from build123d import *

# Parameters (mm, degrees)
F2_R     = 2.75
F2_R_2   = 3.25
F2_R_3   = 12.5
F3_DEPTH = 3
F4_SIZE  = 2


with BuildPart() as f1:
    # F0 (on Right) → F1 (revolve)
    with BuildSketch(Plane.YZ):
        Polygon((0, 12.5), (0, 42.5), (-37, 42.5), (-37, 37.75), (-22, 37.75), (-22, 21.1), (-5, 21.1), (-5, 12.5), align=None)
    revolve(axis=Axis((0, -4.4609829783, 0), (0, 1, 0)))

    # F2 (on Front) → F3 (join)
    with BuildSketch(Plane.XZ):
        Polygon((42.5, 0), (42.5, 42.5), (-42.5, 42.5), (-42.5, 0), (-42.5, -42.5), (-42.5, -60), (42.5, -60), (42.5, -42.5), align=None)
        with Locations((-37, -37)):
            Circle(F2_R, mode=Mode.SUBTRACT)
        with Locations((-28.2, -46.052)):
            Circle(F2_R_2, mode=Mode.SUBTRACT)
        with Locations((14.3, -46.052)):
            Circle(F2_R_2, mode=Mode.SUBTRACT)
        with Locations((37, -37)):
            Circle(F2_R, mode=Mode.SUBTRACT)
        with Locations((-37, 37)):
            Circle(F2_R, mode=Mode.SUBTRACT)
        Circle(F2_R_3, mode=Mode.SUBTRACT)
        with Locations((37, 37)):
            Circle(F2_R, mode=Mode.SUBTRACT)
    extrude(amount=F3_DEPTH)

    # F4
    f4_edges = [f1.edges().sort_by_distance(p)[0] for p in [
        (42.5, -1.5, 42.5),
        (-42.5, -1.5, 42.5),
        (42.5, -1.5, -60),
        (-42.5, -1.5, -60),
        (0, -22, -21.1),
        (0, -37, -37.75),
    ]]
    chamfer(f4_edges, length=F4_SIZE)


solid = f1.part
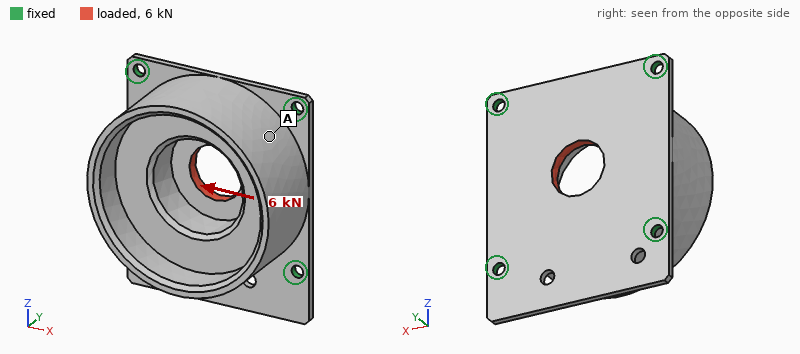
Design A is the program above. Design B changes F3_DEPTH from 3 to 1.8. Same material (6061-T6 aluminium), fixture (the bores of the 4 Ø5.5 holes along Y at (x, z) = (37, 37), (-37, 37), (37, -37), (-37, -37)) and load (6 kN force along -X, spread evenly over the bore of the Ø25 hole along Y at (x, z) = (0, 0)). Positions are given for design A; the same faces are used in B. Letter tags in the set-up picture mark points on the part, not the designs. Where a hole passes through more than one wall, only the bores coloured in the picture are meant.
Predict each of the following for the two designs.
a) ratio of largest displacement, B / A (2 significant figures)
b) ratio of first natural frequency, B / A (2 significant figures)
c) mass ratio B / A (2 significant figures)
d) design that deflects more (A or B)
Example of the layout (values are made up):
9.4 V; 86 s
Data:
1.3; 0.58; 0.97; B
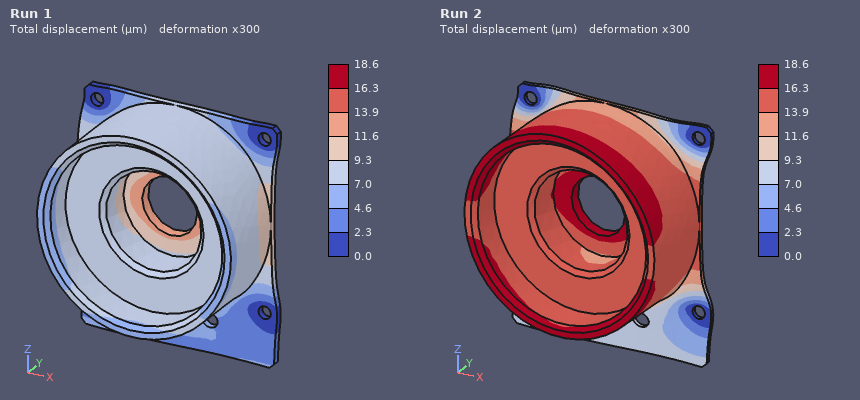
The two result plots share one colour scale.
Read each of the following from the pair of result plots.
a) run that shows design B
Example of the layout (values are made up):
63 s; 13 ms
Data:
Run 2
